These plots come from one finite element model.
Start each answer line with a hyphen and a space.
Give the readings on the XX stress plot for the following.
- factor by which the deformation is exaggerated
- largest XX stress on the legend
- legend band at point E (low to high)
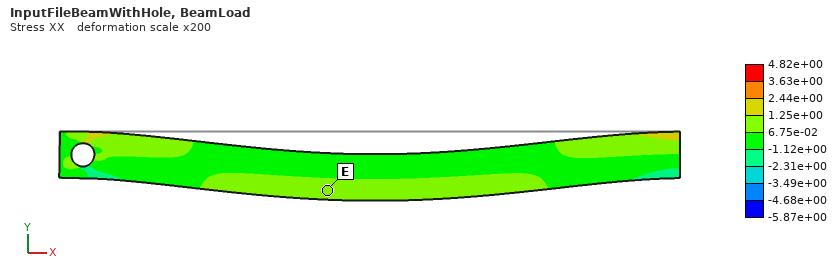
- 200
- 4.82e+00
- 6.75e-02 to 1.25e+00
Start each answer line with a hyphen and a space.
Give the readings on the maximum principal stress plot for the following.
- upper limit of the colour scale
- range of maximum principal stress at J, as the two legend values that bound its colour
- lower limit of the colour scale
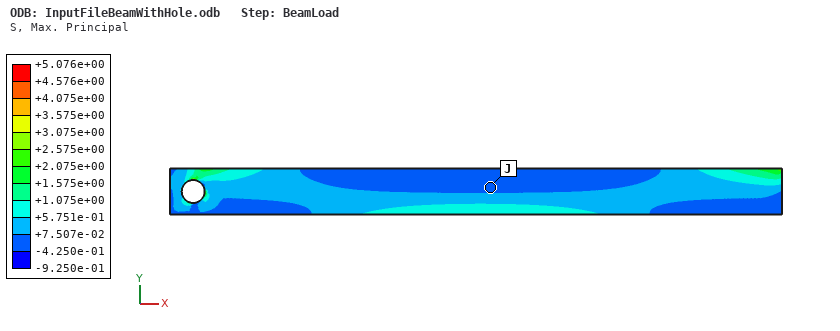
- +5.076e+00
- -4.250e-01 to +7.507e-02
- -9.250e-01
